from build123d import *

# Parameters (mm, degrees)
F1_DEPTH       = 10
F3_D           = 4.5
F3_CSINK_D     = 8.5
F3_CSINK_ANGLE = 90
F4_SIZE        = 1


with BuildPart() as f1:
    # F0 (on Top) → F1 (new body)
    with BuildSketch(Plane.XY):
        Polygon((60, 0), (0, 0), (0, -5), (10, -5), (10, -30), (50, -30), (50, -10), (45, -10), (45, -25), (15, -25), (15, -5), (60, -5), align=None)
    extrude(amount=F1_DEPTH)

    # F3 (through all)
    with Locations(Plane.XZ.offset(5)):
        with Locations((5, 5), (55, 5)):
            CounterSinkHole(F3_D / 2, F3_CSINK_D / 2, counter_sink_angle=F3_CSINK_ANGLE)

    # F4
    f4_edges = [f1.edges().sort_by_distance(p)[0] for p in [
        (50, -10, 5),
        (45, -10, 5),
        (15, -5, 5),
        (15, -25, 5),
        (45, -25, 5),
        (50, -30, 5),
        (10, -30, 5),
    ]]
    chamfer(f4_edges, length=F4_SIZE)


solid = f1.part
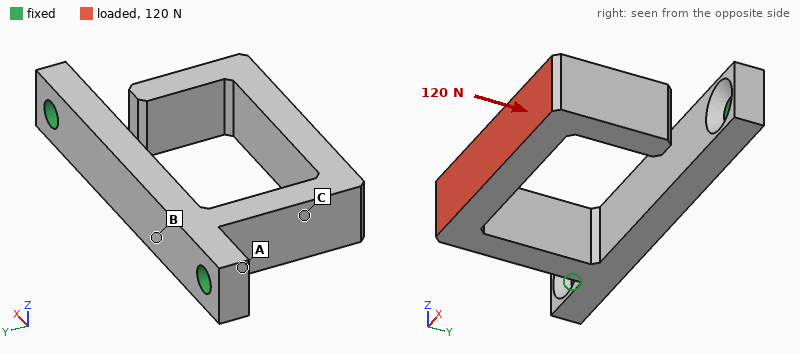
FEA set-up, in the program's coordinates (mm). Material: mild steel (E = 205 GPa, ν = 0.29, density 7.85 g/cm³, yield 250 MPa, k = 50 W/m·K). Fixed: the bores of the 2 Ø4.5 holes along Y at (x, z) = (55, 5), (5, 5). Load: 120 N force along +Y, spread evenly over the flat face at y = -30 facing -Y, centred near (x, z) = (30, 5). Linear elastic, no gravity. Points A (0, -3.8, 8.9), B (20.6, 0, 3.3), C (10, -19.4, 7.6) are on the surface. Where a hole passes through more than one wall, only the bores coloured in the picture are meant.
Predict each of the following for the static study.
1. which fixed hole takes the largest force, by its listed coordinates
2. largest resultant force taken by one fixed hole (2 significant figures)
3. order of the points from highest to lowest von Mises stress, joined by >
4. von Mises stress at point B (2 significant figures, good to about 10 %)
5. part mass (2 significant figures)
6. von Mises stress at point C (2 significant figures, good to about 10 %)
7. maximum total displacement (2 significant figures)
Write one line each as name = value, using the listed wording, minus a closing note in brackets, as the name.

which fixed hole takes the largest force, by its listed coordinates = (5, 5)
largest resultant force taken by one fixed hole = 110 N
order of the points from highest to lowest von Mises stress, joined by > = C > B > A
von Mises stress at point B = 20 MPa
part mass = 51 g
von Mises stress at point C = 48 MPa
maximum total displacement = 0.14 mm
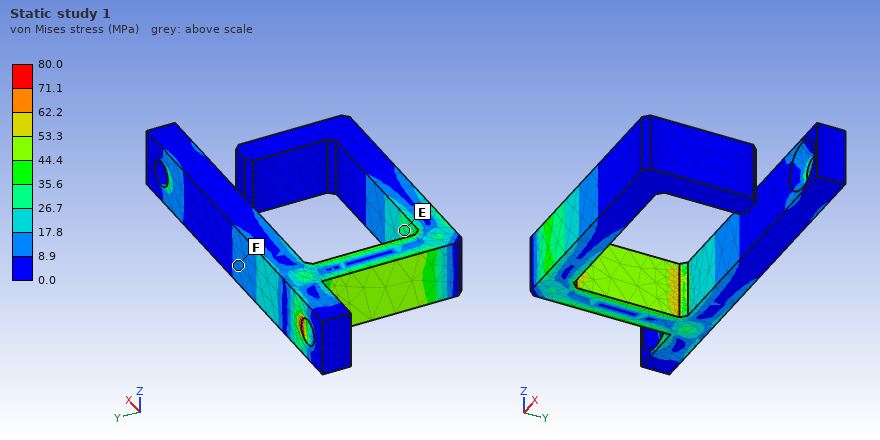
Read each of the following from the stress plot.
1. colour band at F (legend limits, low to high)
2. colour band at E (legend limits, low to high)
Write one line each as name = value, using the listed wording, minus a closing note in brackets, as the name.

colour band at F = 8.9 to 17.8 MPa
colour band at E = 26.7 to 35.6 MPa
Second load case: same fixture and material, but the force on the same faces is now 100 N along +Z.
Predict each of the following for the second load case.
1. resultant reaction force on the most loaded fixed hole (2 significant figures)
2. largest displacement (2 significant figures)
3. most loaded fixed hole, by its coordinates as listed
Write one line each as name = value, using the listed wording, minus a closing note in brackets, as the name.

resultant reaction force on the most loaded fixed hole = 69 N
largest displacement = 91 µm
most loaded fixed hole, by its coordinates as listed = (5, 5)
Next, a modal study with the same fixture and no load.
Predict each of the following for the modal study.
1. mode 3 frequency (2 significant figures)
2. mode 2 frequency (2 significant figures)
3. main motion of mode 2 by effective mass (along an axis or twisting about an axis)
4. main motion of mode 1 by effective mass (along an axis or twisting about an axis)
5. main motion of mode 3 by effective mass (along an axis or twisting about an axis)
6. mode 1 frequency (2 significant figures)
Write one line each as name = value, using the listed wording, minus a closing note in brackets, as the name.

mode 3 frequency = 2700 Hz
mode 2 frequency = 1200 Hz
main motion of mode 2 by effective mass = along Z
main motion of mode 1 by effective mass = along Y
main motion of mode 3 by effective mass = along X
mode 1 frequency = 950 Hz
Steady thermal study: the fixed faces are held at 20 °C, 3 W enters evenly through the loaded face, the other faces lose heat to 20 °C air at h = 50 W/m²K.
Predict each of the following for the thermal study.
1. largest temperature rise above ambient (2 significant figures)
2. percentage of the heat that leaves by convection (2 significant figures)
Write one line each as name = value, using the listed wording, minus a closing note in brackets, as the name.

largest temperature rise above ambient = 24 K
percentage of the heat that leaves by convection = 58 %
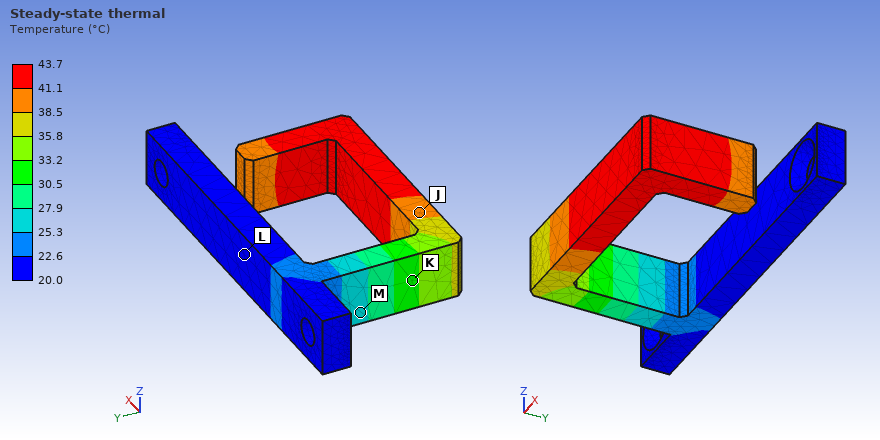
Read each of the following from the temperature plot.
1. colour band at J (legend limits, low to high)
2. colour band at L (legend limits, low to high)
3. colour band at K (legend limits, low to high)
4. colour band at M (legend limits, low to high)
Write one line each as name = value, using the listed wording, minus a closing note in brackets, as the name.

colour band at J = 38.5 to 41.1 °C
colour band at L = 20.0 to 22.6 °C
colour band at K = 30.5 to 33.2 °C
colour band at M = 25.3 to 27.9 °C
